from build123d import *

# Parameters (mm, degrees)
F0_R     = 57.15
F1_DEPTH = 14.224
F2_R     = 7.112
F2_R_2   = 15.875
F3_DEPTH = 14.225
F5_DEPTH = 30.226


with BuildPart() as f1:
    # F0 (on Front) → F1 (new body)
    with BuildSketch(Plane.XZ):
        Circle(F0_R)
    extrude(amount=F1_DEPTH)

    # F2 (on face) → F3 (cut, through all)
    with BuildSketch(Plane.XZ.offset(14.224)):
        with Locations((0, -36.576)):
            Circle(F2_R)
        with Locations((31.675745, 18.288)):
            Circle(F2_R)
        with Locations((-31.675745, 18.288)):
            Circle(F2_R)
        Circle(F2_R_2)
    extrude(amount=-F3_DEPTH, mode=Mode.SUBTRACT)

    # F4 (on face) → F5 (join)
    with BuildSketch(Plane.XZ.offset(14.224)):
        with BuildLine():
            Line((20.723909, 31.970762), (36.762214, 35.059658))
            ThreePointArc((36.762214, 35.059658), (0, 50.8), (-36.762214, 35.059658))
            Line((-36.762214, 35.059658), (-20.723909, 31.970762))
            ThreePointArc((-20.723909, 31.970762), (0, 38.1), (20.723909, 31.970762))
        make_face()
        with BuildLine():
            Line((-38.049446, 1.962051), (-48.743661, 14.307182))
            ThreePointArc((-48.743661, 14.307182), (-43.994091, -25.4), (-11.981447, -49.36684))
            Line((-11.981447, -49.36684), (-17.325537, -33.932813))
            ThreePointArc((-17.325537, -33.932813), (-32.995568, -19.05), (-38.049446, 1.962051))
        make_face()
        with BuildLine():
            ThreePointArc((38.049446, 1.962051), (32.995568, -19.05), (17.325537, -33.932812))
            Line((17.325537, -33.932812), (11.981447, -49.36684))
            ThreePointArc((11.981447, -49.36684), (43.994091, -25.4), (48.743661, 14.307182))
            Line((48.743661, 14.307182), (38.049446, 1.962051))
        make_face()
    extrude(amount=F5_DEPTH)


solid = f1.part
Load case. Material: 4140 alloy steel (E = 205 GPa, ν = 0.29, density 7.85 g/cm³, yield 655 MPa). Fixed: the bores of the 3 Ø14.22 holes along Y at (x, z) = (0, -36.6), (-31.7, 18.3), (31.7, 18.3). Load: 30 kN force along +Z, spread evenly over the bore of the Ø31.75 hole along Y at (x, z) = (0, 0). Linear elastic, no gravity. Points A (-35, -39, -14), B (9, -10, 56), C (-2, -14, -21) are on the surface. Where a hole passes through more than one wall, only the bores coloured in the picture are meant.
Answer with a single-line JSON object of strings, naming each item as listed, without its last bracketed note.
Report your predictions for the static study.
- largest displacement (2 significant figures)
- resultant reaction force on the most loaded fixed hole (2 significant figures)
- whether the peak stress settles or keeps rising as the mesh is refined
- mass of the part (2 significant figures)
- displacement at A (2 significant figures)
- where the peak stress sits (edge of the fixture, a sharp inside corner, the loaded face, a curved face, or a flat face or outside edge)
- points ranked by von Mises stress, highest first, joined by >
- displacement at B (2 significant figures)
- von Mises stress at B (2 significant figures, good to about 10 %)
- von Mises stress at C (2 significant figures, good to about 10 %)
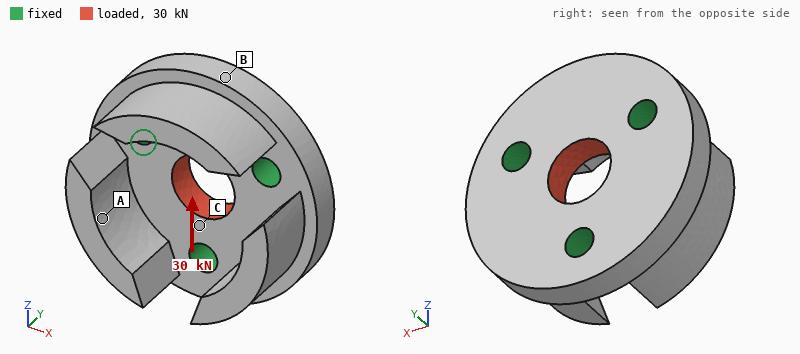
{"largest displacement": "4.3 µm", "resultant reaction force on the most loaded fixed hole": "10 kN", "whether the peak stress settles or keeps rising as the mesh is refined": "keeps rising", "mass of the part": "1.6 kg", "displacement at A": "1.1 µm", "where the peak stress sits": "edge of the fixture", "points ranked by von Mises stress, highest first, joined by >": "C > B > A", "displacement at B": "2.0 µm", "von Mises stress at B": "8.9 MPa", "von Mises stress at C": "27 MPa"}
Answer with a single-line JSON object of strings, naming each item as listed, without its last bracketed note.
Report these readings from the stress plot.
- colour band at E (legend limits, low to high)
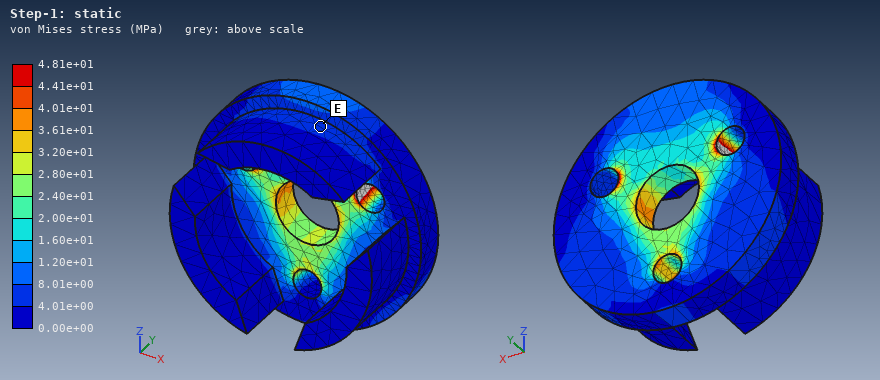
{"colour band at E": "4.01e+00 to 8.01e+00 MPa"}
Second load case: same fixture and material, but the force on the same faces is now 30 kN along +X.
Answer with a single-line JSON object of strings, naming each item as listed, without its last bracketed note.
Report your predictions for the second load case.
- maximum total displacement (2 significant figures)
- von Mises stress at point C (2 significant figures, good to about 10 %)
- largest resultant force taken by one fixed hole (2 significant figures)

{"maximum total displacement": "3.9 µm", "von Mises stress at point C": "23 MPa", "largest resultant force taken by one fixed hole": "10 kN"}
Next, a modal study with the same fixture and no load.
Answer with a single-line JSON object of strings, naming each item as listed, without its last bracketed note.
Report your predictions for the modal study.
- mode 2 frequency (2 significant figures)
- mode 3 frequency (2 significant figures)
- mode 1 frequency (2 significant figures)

{"mode 2 frequency": "4500 Hz", "mode 3 frequency": "4600 Hz", "mode 1 frequency": "4500 Hz"}
